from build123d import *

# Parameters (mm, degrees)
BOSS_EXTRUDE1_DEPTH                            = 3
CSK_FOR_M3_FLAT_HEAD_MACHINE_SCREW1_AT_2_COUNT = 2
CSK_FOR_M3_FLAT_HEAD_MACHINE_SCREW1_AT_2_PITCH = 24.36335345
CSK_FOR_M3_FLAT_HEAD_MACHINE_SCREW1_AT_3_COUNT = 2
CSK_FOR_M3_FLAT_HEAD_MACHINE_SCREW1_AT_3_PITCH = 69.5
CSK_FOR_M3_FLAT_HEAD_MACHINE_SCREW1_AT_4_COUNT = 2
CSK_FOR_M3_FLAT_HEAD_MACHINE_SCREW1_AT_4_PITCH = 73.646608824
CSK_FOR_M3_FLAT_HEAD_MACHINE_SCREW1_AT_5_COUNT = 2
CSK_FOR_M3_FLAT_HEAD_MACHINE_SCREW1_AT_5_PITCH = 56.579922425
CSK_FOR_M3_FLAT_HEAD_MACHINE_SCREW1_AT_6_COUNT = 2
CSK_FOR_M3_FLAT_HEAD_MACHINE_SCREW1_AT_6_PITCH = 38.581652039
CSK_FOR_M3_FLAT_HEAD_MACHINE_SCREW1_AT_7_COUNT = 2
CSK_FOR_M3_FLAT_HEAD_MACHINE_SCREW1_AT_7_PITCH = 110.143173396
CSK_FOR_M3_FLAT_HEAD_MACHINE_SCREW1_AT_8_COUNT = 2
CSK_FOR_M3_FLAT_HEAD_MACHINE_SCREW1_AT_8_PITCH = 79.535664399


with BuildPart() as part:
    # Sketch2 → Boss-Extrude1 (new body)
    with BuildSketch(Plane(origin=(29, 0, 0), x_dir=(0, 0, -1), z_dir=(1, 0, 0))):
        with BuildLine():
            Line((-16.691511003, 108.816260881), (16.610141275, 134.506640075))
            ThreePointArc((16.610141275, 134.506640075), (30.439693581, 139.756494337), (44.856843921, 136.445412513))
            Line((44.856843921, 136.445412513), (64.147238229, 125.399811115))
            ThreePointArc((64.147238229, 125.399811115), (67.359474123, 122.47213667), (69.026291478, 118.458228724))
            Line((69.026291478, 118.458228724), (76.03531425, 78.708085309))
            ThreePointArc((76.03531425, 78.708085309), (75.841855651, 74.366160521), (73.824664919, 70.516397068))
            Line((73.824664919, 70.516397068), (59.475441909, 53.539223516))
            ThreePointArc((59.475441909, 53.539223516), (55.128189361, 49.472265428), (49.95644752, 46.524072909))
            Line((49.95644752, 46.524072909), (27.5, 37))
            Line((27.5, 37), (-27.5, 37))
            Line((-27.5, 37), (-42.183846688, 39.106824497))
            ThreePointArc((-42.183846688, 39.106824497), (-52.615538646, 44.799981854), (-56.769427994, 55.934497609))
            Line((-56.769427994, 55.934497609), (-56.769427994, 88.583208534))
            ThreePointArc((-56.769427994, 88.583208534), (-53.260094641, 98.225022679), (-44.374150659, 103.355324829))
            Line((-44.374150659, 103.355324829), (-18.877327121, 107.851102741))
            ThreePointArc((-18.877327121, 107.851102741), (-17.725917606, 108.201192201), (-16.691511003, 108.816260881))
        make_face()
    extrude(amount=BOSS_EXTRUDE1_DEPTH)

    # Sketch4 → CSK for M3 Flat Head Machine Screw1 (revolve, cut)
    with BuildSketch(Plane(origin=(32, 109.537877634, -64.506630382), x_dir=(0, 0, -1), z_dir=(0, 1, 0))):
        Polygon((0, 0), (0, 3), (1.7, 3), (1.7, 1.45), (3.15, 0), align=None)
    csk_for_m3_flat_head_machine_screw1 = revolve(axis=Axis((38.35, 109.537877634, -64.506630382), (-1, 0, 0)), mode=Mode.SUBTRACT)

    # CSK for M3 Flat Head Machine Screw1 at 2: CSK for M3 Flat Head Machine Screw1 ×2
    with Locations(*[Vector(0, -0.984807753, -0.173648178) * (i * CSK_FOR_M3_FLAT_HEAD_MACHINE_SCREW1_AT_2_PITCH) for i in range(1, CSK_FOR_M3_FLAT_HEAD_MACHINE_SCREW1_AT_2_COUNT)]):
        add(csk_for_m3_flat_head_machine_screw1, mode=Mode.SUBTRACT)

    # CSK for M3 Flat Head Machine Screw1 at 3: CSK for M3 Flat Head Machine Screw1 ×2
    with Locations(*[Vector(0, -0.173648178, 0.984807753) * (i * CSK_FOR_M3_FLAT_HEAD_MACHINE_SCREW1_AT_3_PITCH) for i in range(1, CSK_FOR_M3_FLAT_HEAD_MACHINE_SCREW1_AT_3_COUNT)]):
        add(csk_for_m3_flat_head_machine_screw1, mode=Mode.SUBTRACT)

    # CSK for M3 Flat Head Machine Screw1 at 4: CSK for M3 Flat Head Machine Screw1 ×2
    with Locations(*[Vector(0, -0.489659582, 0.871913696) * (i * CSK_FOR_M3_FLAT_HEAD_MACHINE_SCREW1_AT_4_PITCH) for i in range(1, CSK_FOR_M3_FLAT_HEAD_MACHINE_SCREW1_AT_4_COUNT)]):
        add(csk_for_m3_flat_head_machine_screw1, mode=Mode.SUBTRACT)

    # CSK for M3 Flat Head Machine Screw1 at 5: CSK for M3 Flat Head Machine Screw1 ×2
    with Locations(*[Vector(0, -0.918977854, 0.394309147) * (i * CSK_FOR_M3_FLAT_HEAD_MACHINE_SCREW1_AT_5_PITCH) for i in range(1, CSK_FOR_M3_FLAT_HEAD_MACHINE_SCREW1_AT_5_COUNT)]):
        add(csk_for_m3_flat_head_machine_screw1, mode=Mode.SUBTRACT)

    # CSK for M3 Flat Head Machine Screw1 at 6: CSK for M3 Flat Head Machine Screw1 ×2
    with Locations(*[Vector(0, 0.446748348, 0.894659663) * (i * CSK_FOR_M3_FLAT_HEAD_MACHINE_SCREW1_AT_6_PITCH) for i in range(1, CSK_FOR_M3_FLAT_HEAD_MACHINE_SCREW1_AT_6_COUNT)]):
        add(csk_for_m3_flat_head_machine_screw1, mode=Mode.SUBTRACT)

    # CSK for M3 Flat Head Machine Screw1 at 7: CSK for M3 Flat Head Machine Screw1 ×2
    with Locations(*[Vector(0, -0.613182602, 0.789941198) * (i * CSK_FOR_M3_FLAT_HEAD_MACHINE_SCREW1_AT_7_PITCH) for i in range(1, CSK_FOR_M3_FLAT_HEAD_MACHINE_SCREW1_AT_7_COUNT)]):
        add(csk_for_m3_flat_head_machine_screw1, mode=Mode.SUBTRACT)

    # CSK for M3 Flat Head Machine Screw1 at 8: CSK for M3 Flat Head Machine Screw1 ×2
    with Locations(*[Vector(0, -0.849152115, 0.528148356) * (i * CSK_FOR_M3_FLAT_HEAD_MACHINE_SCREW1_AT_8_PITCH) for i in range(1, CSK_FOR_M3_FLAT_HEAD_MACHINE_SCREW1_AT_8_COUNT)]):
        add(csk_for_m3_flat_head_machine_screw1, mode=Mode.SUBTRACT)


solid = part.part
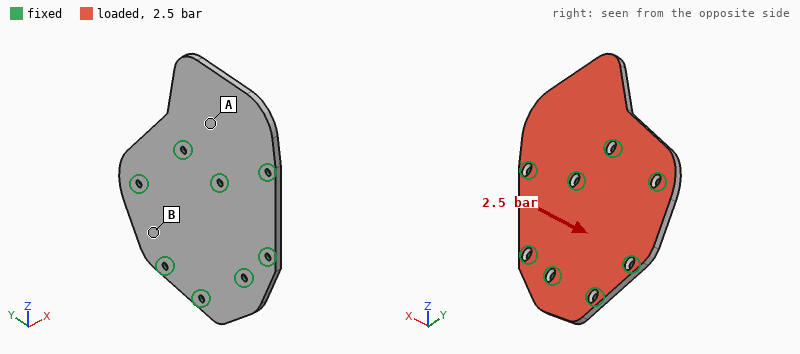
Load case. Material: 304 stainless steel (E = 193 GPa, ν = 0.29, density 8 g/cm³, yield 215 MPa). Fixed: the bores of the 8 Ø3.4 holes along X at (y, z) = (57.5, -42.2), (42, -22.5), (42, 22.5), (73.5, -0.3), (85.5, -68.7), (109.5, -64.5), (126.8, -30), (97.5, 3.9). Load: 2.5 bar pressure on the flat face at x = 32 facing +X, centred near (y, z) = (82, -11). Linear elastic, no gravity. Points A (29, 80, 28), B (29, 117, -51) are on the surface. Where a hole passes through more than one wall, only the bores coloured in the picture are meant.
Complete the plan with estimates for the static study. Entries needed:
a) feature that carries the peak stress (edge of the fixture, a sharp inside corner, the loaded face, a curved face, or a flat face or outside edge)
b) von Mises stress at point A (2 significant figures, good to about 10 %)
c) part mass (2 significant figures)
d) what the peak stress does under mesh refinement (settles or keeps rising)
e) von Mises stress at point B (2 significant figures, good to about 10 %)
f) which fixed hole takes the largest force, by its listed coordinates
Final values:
edge of the fixture
50 MPa
240 g
keeps rising
17 MPa
(97.5, 3.9)
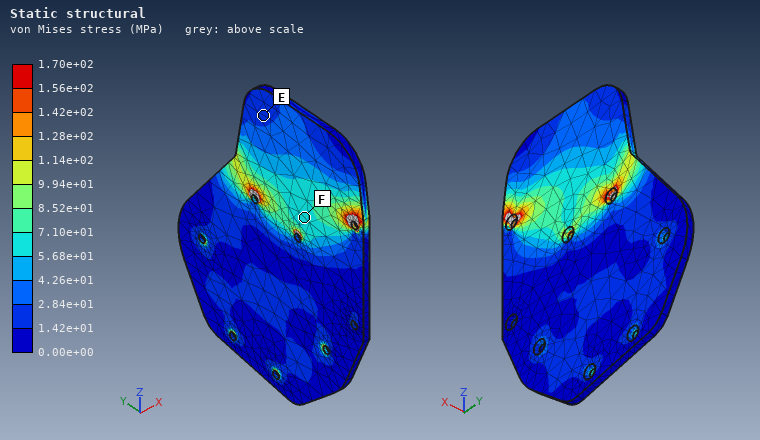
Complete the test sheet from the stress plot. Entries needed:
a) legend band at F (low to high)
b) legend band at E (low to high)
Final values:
5.68e+01 to 7.10e+01 MPa
1.42e+01 to 2.84e+01 MPa
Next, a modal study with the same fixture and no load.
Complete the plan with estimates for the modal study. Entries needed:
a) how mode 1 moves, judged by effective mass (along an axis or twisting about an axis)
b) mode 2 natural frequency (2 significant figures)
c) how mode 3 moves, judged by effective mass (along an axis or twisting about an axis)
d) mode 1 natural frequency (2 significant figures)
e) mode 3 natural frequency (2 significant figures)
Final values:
along X
2800 Hz
along X
1100 Hz
4100 Hz
